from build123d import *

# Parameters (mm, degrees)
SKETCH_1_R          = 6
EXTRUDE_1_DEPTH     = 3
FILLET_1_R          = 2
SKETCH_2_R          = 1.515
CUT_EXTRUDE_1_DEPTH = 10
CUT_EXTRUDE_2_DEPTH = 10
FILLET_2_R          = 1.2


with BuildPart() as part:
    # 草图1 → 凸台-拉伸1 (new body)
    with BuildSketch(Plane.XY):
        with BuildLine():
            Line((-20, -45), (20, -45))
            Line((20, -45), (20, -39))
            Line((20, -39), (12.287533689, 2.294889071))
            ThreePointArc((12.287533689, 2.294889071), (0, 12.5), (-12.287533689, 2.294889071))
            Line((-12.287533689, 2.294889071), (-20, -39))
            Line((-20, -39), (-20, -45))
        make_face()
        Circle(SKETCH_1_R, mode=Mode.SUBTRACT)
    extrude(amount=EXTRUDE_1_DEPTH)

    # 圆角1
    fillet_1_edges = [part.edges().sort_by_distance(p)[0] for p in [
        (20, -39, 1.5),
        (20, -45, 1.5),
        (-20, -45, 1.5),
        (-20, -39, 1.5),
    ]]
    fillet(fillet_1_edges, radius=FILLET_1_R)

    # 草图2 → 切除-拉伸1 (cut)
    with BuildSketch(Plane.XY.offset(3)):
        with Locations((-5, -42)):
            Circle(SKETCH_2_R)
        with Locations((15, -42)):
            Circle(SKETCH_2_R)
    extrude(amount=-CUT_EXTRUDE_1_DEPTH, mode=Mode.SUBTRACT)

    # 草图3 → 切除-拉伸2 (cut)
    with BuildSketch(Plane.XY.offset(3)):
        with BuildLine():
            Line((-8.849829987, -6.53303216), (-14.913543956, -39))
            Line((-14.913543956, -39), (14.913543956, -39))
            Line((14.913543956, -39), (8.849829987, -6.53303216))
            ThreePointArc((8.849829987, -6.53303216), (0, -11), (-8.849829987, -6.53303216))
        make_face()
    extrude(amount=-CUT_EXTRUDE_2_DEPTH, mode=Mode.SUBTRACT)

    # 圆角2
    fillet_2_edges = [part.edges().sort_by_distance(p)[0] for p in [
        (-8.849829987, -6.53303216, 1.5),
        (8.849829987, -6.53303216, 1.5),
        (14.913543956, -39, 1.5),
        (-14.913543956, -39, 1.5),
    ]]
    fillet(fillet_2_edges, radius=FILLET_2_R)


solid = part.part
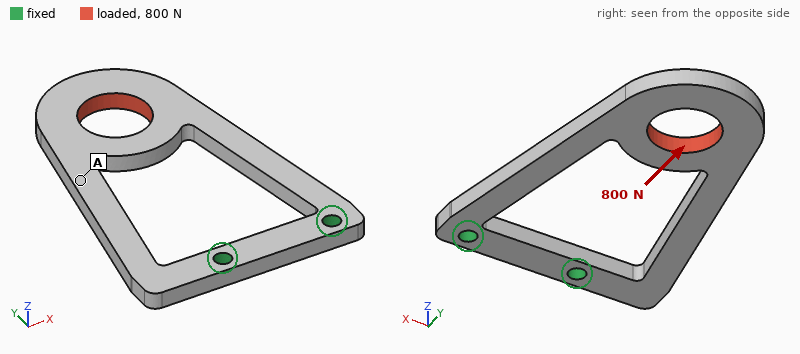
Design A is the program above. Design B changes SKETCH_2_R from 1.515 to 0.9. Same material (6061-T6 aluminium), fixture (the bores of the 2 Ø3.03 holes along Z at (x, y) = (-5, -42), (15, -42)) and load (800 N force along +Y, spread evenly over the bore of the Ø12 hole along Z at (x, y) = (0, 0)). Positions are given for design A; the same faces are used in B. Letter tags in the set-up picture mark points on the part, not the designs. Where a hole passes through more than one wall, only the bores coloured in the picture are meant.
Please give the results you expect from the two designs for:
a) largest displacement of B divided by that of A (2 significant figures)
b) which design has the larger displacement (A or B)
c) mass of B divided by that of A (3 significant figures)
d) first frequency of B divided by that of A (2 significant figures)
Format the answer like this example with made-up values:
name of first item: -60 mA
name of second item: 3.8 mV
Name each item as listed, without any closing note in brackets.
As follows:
largest displacement of B divided by that of A: 1.3
which design has the larger displacement: B
mass of B divided by that of A: 1.01
first frequency of B divided by that of A: 0.98
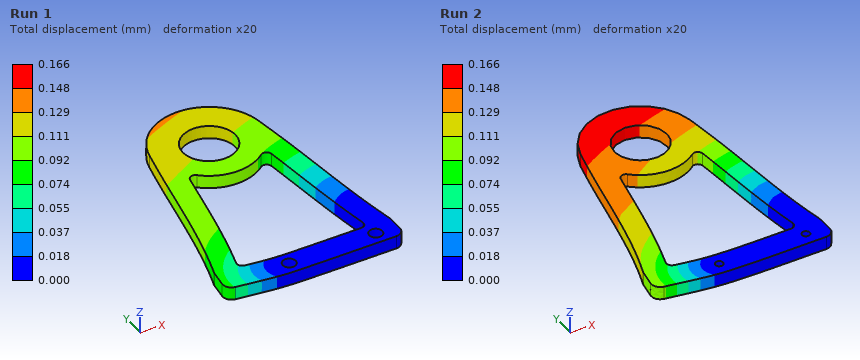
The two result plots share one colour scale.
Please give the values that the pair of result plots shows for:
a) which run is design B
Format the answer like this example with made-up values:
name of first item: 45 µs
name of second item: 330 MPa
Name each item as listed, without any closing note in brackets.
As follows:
which run is design B: Run 2
